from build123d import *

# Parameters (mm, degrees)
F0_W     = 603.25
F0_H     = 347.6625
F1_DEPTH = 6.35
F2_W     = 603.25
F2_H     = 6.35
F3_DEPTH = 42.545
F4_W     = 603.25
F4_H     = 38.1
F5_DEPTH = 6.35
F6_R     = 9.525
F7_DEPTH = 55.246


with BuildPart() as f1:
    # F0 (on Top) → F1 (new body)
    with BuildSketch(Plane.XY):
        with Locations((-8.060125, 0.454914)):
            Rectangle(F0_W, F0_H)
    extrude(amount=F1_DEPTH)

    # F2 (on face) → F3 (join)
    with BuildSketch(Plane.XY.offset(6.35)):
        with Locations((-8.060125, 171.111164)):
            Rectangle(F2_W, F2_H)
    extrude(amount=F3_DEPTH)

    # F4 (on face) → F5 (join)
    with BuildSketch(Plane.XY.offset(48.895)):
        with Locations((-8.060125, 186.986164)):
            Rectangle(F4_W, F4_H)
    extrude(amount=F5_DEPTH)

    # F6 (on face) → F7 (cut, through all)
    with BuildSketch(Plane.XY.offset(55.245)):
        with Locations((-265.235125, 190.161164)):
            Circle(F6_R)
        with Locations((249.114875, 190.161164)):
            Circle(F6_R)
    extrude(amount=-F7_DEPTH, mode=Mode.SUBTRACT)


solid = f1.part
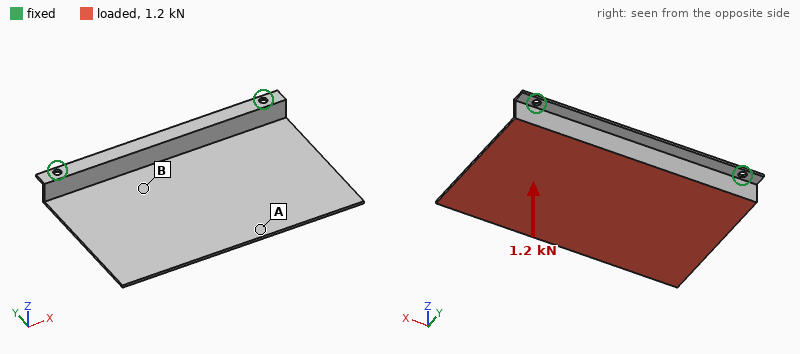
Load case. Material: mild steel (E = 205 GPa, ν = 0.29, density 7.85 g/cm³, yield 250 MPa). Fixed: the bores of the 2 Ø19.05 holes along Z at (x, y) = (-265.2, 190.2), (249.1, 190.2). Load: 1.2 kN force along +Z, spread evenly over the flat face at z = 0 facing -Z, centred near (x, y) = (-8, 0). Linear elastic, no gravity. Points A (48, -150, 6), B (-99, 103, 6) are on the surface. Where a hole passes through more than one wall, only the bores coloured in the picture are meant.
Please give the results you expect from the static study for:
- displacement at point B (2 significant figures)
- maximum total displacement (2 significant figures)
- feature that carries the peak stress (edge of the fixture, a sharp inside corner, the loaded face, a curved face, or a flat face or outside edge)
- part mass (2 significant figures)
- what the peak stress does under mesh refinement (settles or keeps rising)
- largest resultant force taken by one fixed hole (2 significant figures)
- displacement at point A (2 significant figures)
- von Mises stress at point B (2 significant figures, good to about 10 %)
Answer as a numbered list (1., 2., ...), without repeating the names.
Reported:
1. 0.87 mm
2. 5.4 mm
3. edge of the fixture
4. 13 kg
5. keeps rising
6. 1.9 kN
7. 5.0 mm
8. 29 MPa
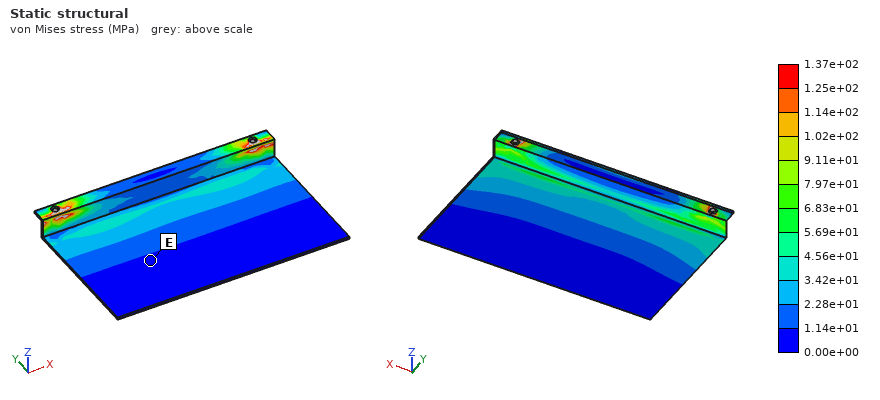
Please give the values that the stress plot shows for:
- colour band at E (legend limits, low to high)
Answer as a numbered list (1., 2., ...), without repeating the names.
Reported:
1. 0.00e+00 to 1.14e+01 MPa
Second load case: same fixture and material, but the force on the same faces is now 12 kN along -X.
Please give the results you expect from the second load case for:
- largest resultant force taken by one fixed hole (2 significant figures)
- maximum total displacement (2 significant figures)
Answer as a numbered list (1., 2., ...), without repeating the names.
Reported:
1. 7.5 kN
2. 1.4 mm
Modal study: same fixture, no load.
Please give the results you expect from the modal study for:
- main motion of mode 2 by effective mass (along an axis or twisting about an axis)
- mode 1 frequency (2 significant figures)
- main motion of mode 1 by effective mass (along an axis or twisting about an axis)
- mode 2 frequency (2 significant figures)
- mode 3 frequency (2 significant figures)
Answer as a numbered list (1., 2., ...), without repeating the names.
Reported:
1. twisting about Y
2. 28 Hz
3. along Z
4. 64 Hz
5. 150 Hz
